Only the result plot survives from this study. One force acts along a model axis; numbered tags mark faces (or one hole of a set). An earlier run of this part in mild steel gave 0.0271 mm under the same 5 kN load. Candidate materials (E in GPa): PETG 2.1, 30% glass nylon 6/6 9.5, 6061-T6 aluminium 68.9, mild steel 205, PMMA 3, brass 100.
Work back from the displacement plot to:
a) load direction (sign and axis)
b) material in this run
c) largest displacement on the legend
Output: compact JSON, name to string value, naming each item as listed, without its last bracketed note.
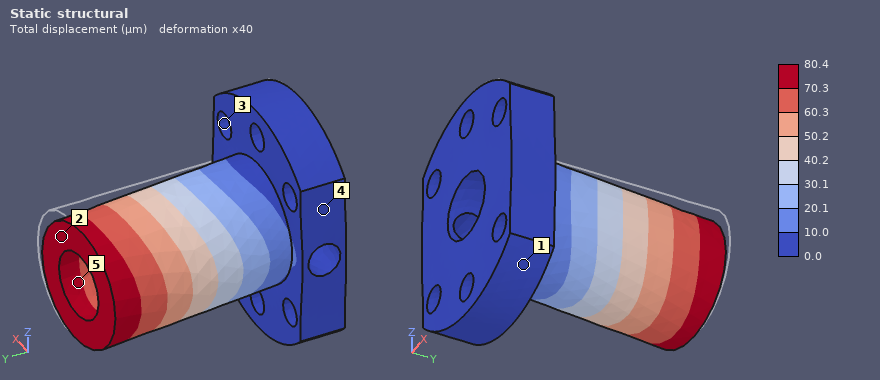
{"load direction": "-X", "material in this run": "6061-T6 aluminium", "largest displacement on the legend": "80.4 µm"}
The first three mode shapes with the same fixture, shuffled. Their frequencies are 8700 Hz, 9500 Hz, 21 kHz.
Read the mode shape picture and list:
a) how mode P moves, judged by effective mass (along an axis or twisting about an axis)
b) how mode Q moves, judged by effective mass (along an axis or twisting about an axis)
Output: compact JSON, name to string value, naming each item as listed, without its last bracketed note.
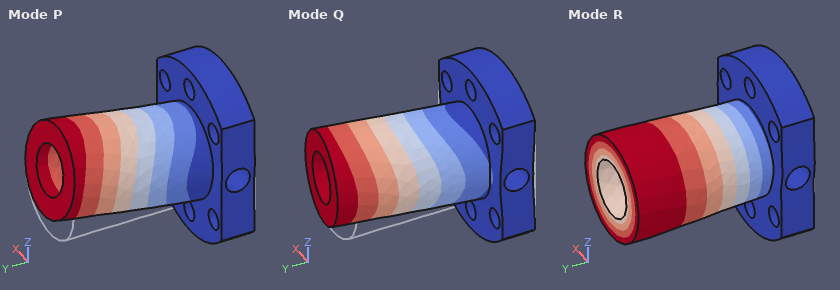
{"how mode P moves, judged by effective mass": "along Z", "how mode Q moves, judged by effective mass": "along X"}
